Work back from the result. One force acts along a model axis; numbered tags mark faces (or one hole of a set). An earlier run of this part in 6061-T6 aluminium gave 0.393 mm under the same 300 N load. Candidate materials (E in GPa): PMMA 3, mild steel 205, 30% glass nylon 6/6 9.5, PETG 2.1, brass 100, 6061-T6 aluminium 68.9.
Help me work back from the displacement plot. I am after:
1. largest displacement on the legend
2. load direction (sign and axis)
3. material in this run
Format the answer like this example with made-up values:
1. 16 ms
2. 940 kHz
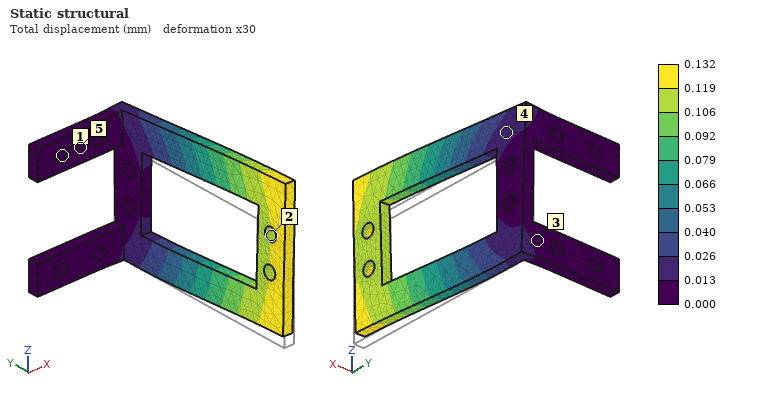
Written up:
1. 0.132 mm
2. +Z
3. mild steel
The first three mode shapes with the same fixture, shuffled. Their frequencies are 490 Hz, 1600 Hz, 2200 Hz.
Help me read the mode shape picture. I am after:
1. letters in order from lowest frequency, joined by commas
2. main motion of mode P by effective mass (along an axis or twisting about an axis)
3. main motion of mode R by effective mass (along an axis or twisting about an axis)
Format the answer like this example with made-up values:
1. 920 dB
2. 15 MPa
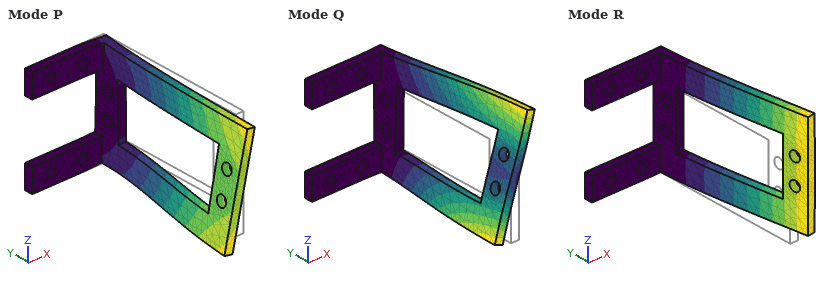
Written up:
1. R, Q, P
2. along Z
3. along X
